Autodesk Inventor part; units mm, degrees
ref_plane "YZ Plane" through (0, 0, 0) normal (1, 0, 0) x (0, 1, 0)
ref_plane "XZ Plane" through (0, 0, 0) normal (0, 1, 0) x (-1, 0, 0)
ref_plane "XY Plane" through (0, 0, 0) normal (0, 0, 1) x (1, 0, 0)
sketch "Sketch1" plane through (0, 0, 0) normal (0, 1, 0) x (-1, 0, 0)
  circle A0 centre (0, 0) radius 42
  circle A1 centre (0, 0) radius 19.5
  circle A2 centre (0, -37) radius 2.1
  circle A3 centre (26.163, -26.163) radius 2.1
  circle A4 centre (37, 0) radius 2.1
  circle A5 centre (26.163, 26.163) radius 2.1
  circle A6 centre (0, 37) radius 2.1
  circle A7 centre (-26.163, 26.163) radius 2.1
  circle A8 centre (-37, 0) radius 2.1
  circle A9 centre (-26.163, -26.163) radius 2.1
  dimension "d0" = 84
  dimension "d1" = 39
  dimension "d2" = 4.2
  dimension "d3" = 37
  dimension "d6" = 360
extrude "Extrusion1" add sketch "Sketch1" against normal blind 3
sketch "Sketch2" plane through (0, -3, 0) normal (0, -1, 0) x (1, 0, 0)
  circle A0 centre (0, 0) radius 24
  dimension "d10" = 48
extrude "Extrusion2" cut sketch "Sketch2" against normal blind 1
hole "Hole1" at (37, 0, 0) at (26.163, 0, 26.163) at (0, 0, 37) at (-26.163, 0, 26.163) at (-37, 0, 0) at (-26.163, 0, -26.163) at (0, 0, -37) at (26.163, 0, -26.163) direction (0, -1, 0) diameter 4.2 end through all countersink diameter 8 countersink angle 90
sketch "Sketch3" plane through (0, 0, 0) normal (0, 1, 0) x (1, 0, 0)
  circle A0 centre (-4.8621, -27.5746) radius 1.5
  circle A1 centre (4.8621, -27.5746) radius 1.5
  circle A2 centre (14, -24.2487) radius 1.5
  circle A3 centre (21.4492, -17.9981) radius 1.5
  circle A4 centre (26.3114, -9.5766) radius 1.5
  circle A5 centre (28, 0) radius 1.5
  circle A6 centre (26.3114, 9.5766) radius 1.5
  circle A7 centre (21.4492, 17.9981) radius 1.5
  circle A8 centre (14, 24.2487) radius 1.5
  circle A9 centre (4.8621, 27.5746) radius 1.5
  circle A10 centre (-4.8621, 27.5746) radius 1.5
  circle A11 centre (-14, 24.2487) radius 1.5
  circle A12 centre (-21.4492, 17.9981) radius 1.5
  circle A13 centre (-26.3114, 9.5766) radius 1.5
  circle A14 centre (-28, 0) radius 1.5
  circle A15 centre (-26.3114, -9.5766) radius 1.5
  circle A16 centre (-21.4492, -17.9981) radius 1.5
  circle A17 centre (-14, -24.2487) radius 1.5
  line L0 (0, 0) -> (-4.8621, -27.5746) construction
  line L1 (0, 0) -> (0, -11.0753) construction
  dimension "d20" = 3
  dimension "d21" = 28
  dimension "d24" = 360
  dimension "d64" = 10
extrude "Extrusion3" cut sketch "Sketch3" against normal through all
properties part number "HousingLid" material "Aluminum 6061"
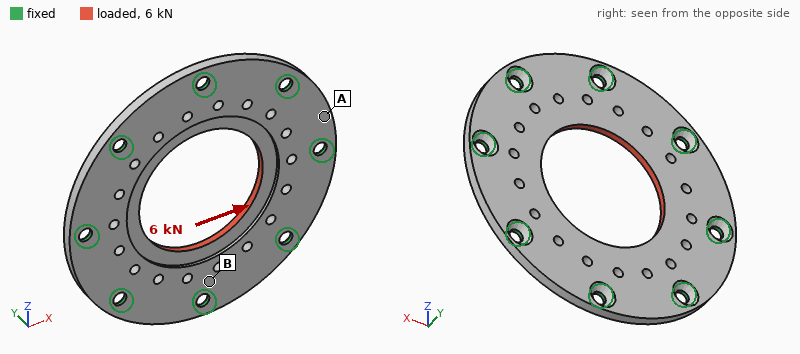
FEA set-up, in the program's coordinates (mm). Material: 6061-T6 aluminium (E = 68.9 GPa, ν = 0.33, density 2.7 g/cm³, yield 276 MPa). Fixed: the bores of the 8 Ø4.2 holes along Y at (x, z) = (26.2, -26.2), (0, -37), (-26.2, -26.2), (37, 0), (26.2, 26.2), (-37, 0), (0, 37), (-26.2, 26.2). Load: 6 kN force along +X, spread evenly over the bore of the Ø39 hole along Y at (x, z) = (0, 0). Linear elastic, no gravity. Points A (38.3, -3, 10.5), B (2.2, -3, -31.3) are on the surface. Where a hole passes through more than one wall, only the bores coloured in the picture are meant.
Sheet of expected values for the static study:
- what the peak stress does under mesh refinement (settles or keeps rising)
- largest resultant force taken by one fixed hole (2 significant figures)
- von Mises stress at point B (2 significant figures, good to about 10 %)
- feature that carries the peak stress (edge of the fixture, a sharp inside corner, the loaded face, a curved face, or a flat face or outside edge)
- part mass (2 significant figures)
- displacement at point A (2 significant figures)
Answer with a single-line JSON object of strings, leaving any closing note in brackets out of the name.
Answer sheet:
{"what the peak stress does under mesh refinement": "keeps rising", "largest resultant force taken by one fixed hole": "1.0 kN", "von Mises stress at point B": "18 MPa", "feature that carries the peak stress": "edge of the fixture", "part mass": "31 g", "displacement at point A": "6.6 µm"}
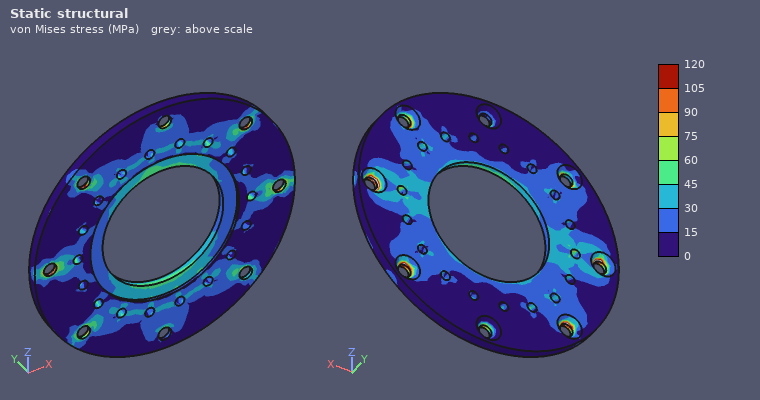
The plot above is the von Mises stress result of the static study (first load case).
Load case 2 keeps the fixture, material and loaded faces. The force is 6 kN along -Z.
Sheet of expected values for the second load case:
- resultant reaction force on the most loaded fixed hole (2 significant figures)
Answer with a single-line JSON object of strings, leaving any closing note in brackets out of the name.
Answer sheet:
{"resultant reaction force on the most loaded fixed hole": "1.0 kN"}
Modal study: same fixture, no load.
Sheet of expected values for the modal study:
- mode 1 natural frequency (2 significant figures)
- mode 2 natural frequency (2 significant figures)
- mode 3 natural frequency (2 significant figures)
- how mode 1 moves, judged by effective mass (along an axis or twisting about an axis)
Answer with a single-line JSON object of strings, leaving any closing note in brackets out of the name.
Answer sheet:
{"mode 1 natural frequency": "7200 Hz", "mode 2 natural frequency": "8500 Hz", "mode 3 natural frequency": "8500 Hz", "how mode 1 moves, judged by effective mass": "along Y"}
